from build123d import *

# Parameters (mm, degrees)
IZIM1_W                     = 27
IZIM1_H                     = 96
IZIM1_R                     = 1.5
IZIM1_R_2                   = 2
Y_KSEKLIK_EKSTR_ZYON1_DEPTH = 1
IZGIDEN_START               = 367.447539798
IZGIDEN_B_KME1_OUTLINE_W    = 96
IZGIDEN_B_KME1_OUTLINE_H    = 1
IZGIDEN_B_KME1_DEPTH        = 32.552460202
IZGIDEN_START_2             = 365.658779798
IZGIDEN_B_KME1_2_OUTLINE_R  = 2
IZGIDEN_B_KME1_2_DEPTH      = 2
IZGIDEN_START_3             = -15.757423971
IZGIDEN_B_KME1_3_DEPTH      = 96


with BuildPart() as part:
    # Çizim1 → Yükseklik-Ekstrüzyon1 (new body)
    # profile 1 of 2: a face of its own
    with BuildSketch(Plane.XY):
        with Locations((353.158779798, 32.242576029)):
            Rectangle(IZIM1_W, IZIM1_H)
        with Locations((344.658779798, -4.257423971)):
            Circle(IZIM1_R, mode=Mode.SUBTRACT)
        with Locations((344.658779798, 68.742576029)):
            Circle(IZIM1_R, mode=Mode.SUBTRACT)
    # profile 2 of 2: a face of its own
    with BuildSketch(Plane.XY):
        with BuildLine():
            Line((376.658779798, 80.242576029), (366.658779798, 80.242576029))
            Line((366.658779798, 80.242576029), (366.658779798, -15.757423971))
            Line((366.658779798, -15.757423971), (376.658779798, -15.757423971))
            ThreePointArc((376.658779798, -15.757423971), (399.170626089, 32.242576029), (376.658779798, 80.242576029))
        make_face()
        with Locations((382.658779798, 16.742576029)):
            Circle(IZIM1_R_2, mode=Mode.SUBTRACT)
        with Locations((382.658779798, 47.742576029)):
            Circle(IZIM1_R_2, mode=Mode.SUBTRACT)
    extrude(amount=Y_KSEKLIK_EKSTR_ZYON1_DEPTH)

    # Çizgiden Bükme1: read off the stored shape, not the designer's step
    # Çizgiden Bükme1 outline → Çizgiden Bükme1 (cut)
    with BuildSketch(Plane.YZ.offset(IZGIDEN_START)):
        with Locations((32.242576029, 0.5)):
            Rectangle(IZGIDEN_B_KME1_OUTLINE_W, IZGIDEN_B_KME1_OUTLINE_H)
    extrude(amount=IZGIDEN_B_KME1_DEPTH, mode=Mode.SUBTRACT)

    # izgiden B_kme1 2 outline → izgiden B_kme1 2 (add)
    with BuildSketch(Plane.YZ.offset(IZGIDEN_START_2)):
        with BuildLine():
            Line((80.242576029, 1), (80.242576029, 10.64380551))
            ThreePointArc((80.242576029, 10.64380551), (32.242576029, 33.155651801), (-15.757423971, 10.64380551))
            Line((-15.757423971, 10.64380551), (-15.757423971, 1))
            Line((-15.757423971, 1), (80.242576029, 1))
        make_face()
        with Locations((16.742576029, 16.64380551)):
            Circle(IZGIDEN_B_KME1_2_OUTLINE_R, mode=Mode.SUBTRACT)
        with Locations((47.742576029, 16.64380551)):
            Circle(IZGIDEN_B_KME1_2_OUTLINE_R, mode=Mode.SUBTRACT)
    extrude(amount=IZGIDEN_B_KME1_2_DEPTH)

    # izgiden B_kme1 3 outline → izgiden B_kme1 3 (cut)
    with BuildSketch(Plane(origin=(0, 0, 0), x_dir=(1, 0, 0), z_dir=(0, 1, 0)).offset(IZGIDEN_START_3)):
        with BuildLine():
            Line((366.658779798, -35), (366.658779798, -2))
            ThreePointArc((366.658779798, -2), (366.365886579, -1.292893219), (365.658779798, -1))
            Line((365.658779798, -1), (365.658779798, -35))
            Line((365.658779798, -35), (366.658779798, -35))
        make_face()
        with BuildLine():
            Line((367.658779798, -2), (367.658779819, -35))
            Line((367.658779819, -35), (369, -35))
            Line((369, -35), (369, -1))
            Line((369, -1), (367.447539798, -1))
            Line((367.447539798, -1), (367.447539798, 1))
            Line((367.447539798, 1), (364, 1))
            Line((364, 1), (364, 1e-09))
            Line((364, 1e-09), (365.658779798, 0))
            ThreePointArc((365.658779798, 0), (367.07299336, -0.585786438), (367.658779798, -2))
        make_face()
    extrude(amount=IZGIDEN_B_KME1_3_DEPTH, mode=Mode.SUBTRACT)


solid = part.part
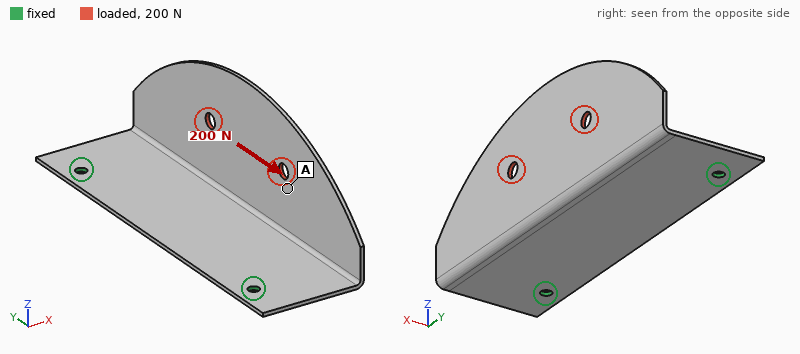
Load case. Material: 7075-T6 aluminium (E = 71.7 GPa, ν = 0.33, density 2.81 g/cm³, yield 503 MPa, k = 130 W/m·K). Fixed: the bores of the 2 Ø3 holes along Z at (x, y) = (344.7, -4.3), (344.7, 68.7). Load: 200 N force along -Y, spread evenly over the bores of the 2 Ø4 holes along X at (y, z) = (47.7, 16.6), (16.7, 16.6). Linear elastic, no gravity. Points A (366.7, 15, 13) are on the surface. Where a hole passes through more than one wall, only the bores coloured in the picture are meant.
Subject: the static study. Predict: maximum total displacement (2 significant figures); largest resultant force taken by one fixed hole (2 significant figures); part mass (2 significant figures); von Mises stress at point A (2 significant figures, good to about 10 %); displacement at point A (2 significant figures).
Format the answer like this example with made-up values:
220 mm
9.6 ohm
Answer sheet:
0.89 mm
120 N
14 g
34 MPa
0.38 mm
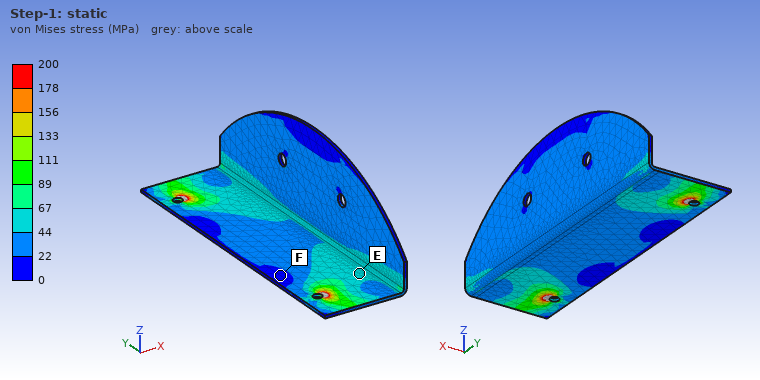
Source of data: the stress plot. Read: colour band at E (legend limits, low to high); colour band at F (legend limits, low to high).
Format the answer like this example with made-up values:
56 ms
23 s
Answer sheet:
44 to 67 MPa
0 to 22 MPa
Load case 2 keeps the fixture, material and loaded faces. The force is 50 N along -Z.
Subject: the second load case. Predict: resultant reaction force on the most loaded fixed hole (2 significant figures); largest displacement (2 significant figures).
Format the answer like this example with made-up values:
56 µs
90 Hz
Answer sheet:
25 N
1.2 mm
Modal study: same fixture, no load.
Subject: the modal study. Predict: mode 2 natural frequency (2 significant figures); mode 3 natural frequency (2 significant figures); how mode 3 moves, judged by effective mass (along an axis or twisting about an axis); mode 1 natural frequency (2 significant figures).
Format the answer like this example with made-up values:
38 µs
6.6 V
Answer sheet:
760 Hz
890 Hz
along Z
370 Hz
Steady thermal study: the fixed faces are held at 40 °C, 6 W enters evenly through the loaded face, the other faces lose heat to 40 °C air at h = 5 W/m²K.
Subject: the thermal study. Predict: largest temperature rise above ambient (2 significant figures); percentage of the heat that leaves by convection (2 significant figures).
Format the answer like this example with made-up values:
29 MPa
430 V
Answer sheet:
33 K
15 %
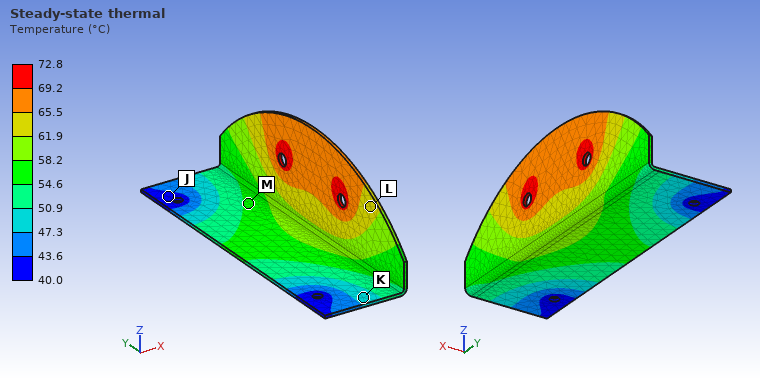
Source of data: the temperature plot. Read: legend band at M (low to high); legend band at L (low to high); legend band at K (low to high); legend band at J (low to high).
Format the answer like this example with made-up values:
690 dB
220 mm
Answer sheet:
54.6 to 58.2 °C
61.9 to 65.5 °C
47.3 to 50.9 °C
40.0 to 43.6 °C
